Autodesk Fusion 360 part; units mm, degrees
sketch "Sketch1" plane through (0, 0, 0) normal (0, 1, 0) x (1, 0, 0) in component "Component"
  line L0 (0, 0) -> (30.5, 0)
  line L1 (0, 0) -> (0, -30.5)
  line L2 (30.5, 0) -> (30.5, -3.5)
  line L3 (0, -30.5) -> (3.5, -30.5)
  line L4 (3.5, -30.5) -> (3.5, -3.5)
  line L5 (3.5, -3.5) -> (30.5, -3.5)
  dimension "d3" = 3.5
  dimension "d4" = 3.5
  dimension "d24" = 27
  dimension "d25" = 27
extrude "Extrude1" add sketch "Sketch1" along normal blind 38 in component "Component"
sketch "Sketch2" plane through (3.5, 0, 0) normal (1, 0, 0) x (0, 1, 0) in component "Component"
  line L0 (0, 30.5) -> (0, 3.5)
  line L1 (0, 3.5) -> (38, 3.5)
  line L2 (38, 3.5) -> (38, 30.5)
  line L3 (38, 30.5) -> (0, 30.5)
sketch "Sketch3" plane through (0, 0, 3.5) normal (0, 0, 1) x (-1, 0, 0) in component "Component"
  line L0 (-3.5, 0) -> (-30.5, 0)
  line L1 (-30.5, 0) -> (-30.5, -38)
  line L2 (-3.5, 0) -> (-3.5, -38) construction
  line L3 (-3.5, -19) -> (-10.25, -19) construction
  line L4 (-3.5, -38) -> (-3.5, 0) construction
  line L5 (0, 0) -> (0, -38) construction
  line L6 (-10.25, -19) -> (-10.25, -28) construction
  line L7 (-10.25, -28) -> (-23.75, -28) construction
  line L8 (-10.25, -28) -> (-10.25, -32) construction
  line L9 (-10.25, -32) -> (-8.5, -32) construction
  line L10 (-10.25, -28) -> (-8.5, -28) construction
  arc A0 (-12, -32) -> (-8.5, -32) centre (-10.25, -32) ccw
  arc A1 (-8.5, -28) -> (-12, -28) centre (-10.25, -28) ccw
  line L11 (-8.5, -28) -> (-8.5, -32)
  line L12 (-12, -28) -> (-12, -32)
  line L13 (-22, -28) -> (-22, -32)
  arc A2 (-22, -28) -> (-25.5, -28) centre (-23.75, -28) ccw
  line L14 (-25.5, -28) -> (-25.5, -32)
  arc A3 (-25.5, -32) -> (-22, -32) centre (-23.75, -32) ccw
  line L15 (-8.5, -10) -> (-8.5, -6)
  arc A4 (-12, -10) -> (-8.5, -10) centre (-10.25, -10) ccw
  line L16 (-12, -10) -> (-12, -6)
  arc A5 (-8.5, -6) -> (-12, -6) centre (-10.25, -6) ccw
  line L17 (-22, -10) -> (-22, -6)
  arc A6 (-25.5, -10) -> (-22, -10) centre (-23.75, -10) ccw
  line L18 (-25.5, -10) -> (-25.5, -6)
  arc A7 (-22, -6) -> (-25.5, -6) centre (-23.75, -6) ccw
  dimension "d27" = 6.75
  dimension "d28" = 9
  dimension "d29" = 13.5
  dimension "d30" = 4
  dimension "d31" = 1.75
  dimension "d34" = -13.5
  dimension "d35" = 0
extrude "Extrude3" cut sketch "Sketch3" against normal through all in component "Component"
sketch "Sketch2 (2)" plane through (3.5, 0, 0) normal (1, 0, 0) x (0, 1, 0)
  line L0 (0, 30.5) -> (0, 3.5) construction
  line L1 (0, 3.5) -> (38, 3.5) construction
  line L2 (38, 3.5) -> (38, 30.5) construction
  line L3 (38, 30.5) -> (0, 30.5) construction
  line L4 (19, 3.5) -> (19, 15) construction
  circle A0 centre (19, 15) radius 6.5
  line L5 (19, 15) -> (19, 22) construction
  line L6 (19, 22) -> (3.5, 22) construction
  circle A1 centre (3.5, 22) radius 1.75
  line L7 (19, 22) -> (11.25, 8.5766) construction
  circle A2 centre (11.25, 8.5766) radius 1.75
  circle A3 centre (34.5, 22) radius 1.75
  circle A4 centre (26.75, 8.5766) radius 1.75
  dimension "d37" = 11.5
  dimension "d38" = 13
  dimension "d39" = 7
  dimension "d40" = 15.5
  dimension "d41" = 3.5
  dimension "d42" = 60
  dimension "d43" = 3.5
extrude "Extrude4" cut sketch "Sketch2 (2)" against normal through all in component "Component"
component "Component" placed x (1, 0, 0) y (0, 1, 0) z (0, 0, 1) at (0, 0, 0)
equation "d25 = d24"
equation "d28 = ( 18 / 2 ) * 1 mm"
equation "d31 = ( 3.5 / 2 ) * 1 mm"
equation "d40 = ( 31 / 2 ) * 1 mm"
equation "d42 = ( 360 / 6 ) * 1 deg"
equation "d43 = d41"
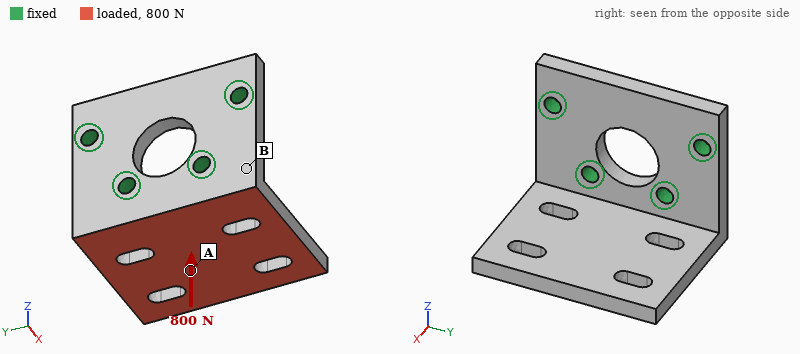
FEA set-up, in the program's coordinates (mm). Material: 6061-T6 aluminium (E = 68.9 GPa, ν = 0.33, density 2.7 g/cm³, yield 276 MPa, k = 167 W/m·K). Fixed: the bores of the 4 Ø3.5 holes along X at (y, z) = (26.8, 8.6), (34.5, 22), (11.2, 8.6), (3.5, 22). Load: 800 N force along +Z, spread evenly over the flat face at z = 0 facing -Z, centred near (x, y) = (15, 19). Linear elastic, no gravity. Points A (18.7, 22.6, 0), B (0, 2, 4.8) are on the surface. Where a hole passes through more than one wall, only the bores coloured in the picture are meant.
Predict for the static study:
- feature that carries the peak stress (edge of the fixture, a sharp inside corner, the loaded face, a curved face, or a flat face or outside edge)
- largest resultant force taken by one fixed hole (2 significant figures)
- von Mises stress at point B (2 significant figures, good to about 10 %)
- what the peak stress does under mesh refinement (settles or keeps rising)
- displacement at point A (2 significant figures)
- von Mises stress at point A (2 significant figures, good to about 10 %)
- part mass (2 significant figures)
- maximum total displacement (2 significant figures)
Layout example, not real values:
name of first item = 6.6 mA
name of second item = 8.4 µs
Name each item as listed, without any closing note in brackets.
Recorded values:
feature that carries the peak stress = edge of the fixture
largest resultant force taken by one fixed hole = 370 N
von Mises stress at point B = 98 MPa
what the peak stress does under mesh refinement = keeps rising
displacement at point A = 0.25 mm
von Mises stress at point A = 27 MPa
part mass = 18 g
maximum total displacement = 0.48 mm
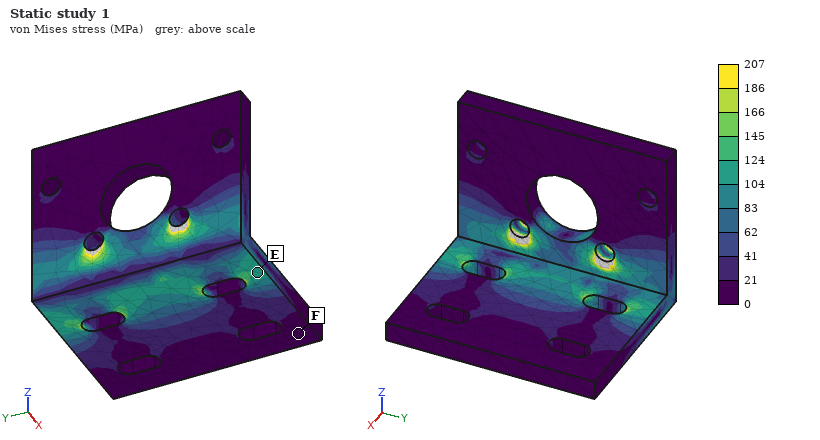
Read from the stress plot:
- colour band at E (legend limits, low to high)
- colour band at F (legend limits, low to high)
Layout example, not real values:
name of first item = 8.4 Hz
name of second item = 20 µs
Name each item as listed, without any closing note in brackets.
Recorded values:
colour band at E = 104 to 124 MPa
colour band at F = 0 to 21 MPa
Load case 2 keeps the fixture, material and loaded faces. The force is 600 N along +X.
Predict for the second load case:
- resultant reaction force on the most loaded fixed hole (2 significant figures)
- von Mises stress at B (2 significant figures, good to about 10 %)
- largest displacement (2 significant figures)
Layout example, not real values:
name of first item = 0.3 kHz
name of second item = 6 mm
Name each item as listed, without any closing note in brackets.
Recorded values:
resultant reaction force on the most loaded fixed hole = 340 N
von Mises stress at B = 23 MPa
largest displacement = 0.10 mm
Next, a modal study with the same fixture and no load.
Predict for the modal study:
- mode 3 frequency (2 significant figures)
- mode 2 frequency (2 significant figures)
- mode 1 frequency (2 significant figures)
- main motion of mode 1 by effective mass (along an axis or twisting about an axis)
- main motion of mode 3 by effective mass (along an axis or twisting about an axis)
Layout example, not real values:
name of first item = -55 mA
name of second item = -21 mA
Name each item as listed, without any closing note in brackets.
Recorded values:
mode 3 frequency = 7700 Hz
mode 2 frequency = 5400 Hz
mode 1 frequency = 2500 Hz
main motion of mode 1 by effective mass = along Z
main motion of mode 3 by effective mass = along Y
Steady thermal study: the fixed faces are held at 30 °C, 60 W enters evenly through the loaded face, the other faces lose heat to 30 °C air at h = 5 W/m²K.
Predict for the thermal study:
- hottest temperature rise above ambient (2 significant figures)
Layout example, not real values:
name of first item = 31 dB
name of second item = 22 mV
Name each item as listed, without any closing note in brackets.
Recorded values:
hottest temperature rise above ambient = 65 K
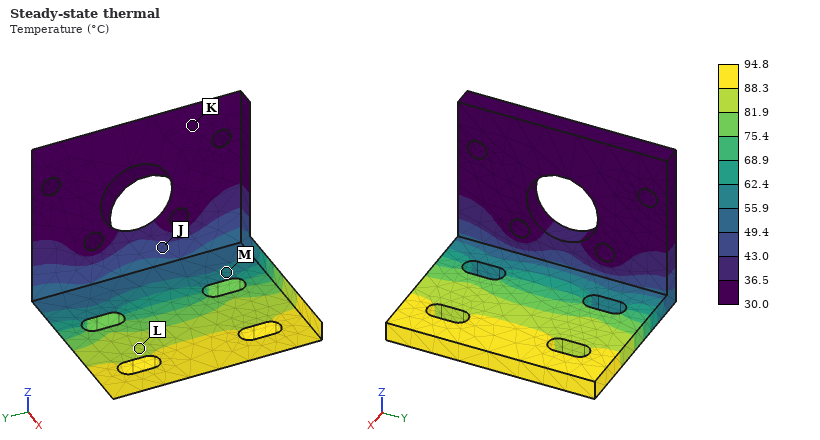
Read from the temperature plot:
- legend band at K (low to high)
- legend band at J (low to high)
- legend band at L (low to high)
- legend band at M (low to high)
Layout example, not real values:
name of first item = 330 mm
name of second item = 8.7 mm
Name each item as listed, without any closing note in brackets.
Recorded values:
legend band at K = 30.0 to 36.5 °C
legend band at J = 43.0 to 49.4 °C
legend band at L = 81.9 to 88.3 °C
legend band at M = 55.9 to 62.4 °C
